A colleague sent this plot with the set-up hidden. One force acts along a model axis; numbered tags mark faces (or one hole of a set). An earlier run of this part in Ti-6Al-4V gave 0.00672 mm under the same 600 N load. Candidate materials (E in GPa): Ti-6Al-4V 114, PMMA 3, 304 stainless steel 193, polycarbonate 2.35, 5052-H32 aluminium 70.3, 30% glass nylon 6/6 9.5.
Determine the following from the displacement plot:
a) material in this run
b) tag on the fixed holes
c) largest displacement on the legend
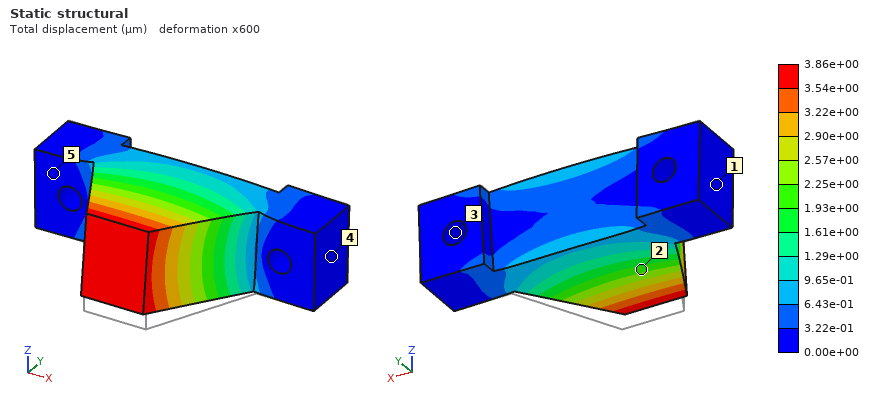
304 stainless steel
3
3.86e+00 µm
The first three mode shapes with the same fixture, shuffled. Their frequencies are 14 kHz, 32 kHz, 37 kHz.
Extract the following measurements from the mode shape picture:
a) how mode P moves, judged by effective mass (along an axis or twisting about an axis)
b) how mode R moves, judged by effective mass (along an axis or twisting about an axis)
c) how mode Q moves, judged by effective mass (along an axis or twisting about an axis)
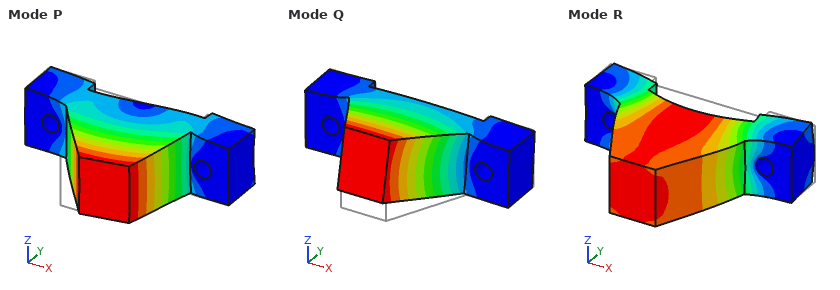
along X
along Y
along Z
